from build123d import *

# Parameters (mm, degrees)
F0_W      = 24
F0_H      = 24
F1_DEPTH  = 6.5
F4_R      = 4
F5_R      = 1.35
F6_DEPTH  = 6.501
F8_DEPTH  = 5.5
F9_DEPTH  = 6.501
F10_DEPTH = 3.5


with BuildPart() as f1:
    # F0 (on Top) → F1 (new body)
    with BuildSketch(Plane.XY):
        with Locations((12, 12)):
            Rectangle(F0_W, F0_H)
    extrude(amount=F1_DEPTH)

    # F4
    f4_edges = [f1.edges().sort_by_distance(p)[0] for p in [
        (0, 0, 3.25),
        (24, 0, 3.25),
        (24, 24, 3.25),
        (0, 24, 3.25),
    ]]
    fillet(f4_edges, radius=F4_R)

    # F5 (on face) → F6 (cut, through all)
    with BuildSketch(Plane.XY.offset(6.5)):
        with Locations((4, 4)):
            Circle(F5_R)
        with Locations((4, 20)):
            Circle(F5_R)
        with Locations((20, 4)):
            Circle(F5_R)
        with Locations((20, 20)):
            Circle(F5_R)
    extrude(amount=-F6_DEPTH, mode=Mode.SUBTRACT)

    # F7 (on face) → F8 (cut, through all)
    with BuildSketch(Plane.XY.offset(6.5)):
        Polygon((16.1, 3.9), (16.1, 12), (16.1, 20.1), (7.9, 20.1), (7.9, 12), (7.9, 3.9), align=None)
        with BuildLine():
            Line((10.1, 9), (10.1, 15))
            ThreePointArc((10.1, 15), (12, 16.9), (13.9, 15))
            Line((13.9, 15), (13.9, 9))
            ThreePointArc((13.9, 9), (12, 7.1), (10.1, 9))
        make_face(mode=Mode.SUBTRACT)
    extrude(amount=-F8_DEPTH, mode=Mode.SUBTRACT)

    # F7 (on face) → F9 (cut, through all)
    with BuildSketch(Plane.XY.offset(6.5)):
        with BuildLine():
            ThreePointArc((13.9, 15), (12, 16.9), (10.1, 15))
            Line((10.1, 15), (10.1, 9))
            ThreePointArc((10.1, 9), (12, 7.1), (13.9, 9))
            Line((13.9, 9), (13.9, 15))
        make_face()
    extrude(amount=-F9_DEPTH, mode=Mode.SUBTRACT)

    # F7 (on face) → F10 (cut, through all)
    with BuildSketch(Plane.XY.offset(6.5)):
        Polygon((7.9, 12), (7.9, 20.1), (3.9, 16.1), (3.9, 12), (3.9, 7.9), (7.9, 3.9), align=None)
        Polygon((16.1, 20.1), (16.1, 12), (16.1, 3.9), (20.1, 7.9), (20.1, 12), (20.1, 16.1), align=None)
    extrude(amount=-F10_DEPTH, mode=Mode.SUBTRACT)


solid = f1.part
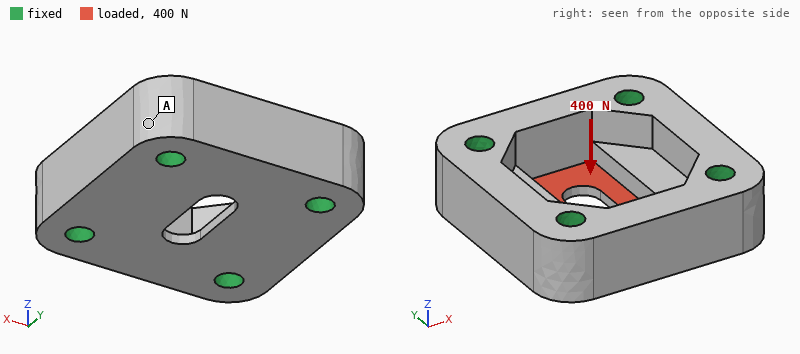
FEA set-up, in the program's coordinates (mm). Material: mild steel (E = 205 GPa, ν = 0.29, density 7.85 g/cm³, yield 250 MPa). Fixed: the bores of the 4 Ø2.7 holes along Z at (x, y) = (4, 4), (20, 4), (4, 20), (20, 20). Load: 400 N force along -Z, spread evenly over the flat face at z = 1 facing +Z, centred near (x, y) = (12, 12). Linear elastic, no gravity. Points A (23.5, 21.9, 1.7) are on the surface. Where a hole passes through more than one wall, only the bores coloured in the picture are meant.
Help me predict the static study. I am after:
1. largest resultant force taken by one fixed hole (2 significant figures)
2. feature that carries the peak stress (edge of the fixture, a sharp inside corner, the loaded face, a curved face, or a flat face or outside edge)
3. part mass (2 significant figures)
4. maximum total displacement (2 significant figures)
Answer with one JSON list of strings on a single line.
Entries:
["100 N", "a curved face", "19 g", "3.3 µm"]
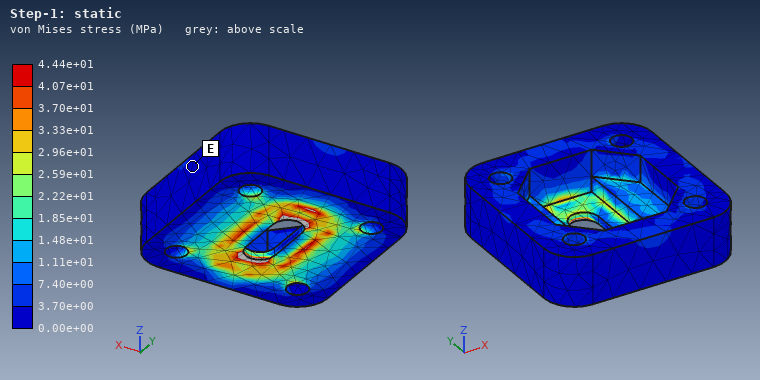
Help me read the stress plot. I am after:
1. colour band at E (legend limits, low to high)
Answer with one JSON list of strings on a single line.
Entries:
["0.00e+00 to 3.70e+00 MPa"]
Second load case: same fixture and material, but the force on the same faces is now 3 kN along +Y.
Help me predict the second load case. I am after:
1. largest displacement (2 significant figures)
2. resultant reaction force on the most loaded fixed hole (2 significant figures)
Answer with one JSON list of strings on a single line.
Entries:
["4.1 µm", "770 N"]
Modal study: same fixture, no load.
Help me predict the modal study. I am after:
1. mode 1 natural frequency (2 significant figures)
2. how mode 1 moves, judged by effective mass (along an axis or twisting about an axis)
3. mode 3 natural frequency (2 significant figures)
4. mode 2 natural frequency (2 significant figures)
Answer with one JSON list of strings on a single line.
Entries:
["64 kHz", "along Z", "77 kHz", "67 kHz"]
